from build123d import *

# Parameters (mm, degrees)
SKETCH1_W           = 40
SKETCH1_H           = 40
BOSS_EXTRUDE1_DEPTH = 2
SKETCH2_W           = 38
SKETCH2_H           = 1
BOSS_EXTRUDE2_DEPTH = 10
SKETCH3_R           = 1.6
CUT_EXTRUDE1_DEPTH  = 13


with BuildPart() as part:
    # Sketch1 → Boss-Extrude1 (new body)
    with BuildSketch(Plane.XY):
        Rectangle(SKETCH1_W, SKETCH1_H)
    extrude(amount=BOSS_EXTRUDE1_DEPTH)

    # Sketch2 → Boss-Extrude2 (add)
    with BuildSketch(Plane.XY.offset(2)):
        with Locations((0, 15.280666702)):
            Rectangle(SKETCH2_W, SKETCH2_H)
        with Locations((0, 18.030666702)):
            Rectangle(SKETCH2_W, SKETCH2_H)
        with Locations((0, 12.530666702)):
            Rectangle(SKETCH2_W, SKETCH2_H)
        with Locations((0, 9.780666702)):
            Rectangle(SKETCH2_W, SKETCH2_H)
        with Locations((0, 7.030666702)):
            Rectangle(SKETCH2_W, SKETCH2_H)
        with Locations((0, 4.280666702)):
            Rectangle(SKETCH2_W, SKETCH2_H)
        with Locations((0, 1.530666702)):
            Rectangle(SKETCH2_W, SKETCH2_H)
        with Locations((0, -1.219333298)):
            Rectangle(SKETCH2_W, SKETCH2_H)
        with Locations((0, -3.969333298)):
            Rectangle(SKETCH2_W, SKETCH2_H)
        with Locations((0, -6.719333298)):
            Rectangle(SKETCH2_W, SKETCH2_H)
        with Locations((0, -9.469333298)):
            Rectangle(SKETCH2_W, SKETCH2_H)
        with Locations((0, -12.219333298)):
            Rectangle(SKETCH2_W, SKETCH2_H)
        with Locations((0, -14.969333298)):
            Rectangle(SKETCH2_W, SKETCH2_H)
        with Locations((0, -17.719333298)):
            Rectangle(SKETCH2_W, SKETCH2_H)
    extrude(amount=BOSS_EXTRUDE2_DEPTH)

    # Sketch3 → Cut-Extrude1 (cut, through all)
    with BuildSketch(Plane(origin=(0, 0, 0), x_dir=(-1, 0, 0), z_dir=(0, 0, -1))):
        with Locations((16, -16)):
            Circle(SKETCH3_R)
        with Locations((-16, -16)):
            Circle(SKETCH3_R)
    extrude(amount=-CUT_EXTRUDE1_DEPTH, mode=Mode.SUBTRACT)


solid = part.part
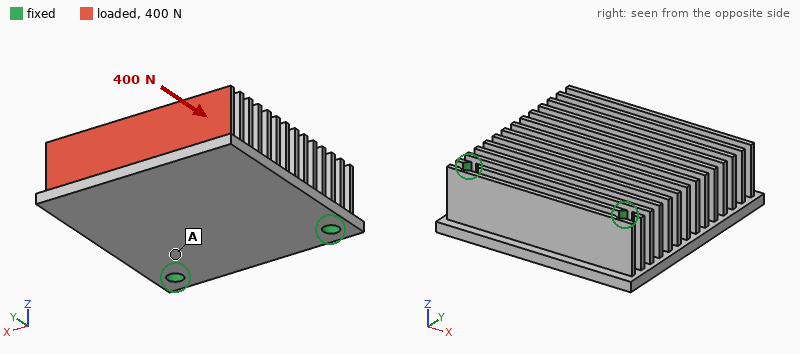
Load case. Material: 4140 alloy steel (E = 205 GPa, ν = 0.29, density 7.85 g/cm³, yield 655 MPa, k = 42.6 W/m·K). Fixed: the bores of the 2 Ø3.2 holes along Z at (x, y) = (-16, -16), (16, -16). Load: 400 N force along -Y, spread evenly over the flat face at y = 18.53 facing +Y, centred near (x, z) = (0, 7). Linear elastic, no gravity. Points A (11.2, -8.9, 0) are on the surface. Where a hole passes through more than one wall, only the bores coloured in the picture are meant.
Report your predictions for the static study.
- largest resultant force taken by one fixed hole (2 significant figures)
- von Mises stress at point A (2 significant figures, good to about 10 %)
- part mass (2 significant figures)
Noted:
200 N
71 MPa
66 g
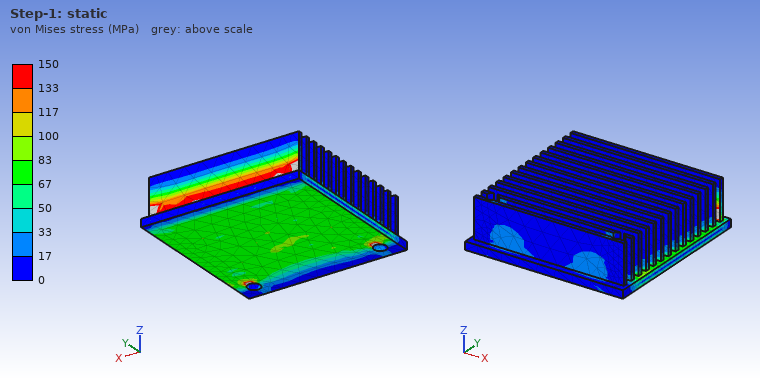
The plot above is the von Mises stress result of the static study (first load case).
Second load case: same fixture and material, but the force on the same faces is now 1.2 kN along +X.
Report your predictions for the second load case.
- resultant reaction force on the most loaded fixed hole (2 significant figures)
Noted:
1.4 kN
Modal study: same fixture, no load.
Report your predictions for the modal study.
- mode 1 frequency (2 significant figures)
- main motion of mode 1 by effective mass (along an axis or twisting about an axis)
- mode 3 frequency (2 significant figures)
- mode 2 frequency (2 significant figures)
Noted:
800 Hz
along Z
3800 Hz
2000 Hz
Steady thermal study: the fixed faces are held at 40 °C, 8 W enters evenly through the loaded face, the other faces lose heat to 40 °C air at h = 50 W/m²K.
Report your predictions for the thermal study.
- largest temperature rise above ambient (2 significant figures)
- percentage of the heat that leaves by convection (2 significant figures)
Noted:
52 K
86 %
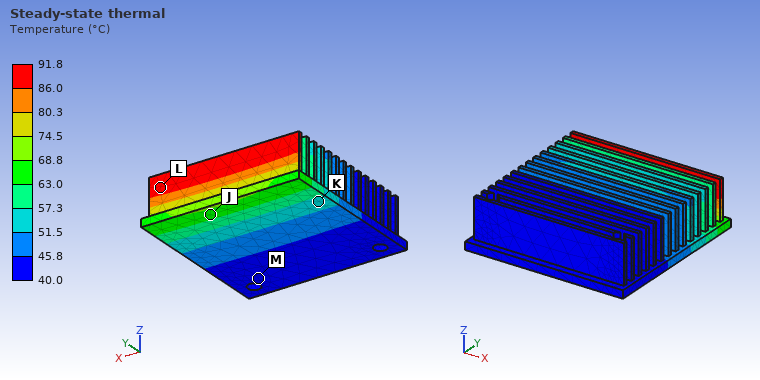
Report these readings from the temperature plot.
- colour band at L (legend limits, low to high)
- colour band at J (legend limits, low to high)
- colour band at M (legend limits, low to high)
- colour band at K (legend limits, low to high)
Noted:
86.0 to 91.8 °C
63.0 to 68.8 °C
40.0 to 45.8 °C
51.5 to 57.3 °C
